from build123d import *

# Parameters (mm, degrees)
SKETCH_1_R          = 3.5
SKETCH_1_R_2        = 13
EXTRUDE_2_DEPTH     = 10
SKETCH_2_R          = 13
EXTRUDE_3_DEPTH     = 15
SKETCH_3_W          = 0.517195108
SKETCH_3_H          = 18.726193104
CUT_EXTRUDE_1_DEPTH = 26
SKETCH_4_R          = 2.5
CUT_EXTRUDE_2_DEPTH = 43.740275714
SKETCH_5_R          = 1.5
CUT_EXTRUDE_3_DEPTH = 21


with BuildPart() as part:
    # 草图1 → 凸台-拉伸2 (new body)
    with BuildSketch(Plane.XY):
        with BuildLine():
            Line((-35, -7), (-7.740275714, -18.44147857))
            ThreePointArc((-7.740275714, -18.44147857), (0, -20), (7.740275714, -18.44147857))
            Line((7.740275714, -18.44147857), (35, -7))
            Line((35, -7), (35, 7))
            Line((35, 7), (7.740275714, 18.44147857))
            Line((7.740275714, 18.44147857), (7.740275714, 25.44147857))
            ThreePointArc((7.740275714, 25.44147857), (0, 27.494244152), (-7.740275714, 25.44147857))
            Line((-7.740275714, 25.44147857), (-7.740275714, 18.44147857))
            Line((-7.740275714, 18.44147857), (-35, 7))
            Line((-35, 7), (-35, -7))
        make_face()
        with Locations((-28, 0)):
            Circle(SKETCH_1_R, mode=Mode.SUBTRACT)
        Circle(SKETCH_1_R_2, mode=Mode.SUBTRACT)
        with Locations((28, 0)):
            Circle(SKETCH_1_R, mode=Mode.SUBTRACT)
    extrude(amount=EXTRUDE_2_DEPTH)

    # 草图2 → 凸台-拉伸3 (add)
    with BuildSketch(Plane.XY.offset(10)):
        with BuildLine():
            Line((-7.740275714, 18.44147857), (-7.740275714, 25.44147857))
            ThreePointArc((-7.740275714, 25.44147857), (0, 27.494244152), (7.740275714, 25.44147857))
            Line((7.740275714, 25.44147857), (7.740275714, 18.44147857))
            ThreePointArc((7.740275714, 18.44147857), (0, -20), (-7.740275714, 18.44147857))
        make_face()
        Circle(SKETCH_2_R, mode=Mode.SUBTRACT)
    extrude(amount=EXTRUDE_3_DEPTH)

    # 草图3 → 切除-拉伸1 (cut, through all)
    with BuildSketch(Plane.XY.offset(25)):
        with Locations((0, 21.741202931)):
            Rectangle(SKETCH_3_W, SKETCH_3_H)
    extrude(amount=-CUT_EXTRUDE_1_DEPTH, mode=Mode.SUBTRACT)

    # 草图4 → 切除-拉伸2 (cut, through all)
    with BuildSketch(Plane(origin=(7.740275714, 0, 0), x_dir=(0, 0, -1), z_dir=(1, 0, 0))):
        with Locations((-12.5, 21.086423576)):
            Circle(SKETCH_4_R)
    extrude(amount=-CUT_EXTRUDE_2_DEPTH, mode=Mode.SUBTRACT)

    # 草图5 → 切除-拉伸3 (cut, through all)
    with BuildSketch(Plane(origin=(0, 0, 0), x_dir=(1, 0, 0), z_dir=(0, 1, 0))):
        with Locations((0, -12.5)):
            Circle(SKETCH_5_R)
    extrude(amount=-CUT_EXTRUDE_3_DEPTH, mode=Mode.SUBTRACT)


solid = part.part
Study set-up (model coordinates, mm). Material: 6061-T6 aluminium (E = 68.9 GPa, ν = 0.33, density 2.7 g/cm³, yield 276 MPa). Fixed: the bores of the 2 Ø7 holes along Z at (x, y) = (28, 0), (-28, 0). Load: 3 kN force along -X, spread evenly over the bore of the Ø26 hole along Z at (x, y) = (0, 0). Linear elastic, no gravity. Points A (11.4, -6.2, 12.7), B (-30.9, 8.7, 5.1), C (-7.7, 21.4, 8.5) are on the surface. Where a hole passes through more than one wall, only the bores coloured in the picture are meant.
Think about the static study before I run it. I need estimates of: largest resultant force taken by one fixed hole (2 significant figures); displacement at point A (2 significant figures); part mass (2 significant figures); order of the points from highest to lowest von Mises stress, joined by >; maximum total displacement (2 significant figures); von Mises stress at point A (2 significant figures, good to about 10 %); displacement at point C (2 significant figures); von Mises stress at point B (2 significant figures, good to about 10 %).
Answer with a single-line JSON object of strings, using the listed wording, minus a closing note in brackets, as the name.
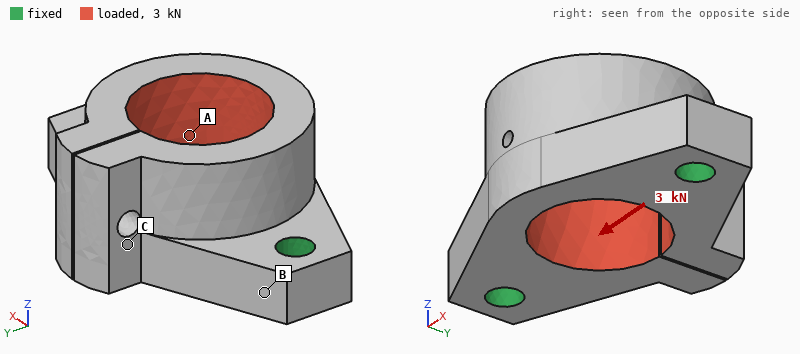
{"largest resultant force taken by one fixed hole": "1.5 kN", "displacement at point A": "4.6 µm", "part mass": "73 g", "order of the points from highest to lowest von Mises stress, joined by >": "A > B > C", "maximum total displacement": "29 µm", "von Mises stress at point A": "13 MPa", "displacement at point C": "15 µm", "von Mises stress at point B": "6.3 MPa"}
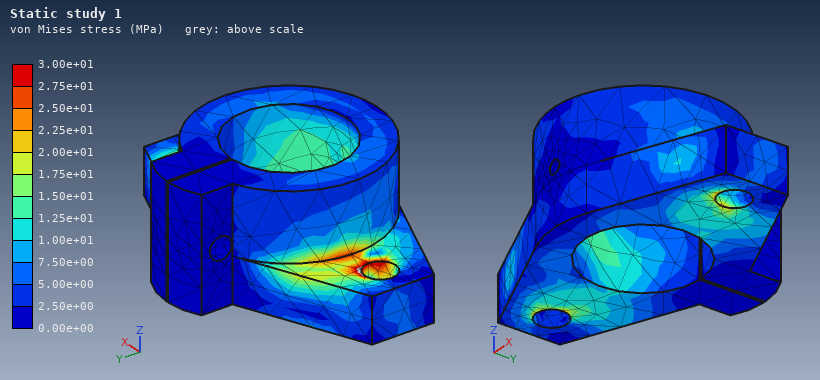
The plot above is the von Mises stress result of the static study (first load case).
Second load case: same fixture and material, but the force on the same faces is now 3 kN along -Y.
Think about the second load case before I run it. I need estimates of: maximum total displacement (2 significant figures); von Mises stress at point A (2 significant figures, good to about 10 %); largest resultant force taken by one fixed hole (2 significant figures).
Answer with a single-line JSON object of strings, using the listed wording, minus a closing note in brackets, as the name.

{"maximum total displacement": "50 µm", "von Mises stress at point A": "6.2 MPa", "largest resultant force taken by one fixed hole": "1.8 kN"}
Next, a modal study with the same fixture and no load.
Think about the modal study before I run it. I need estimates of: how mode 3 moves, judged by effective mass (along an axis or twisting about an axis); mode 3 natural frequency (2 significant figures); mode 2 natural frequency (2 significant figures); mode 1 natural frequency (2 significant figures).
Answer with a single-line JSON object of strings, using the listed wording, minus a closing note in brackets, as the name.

{"how mode 3 moves, judged by effective mass": "along Y", "mode 3 natural frequency": "6200 Hz", "mode 2 natural frequency": "5600 Hz", "mode 1 natural frequency": "5600 Hz"}
